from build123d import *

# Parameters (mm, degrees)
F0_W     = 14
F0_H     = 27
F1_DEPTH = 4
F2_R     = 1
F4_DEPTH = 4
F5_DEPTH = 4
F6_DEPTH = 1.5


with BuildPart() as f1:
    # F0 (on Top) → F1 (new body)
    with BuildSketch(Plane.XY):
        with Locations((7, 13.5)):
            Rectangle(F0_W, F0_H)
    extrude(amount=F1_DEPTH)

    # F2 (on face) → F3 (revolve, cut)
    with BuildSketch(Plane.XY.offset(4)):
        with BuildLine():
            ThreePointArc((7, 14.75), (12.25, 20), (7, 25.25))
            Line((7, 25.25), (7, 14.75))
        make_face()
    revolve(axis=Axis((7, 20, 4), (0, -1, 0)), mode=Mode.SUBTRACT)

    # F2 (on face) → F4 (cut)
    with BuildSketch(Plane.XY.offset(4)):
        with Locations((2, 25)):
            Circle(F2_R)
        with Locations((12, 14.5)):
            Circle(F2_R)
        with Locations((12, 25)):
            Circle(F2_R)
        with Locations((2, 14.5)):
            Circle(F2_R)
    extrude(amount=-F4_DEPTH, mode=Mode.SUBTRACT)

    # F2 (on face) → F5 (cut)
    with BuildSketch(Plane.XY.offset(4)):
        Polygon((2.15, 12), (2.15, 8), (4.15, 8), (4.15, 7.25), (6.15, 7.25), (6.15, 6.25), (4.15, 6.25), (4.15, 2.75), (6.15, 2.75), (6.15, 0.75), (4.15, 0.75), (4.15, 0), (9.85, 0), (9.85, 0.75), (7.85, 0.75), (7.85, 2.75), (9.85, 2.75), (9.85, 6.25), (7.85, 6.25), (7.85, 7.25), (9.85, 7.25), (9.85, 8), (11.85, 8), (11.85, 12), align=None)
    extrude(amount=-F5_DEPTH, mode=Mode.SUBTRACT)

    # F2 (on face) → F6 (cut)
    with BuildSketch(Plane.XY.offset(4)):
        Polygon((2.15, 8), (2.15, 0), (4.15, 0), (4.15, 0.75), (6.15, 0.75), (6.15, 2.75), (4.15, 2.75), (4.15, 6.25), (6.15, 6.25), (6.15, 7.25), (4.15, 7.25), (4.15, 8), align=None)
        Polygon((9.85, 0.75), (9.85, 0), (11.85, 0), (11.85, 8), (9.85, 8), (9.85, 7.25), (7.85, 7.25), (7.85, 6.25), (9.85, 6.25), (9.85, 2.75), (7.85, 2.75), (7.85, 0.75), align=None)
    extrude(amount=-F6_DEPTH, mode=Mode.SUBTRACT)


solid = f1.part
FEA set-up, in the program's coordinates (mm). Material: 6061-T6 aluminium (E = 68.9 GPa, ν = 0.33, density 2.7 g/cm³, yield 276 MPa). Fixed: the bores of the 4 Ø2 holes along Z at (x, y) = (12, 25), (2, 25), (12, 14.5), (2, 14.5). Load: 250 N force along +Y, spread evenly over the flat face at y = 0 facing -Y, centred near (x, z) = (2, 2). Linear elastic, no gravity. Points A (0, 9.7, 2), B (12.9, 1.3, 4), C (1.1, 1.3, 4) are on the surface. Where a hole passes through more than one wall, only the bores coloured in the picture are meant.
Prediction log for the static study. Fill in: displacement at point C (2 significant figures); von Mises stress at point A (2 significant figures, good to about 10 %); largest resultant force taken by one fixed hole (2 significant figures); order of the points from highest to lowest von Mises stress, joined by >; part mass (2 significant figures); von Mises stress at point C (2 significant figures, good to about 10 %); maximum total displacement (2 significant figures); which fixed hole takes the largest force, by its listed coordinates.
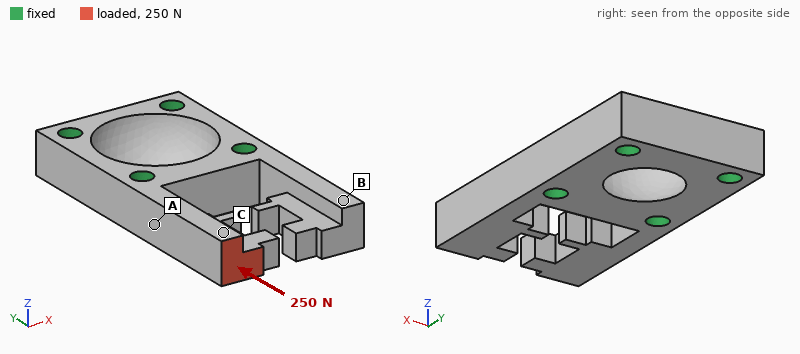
39 µm
29 MPa
250 N
A > C > B
2.2 g
18 MPa
52 µm
(2, 14.5)
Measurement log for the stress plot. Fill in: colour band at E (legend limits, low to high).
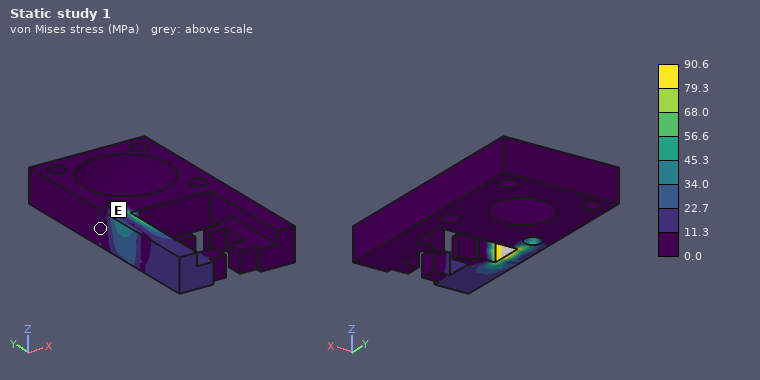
0.0 to 11.3 MPa
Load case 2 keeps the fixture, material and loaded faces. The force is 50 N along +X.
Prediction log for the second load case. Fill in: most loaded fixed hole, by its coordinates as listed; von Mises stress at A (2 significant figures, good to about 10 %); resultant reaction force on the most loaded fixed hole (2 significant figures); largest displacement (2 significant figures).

(12, 14.5)
150 MPa
47 N
0.15 mm
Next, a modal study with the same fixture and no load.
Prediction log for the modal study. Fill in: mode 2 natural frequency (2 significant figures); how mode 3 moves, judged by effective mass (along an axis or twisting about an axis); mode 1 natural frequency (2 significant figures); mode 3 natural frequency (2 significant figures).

7400 Hz
along Z
7400 Hz
12 kHz
